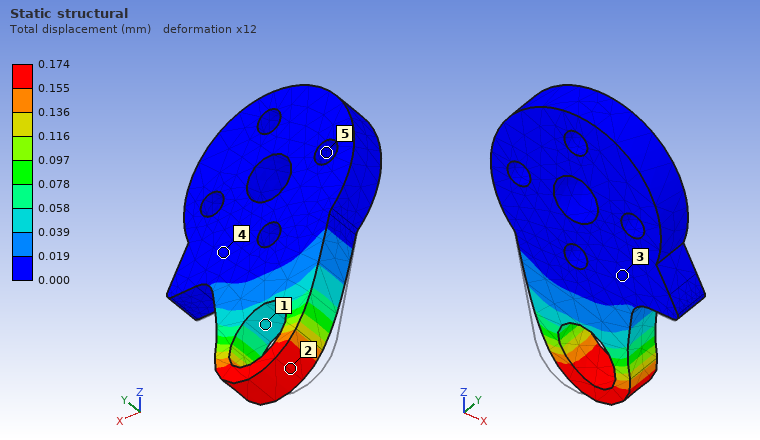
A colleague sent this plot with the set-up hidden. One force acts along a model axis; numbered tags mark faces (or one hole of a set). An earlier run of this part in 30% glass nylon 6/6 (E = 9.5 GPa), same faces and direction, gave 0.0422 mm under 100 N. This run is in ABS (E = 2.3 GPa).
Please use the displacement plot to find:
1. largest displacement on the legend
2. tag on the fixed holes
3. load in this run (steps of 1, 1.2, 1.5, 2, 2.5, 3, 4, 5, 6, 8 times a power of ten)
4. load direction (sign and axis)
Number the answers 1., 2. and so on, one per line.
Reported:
1. 0.174 mm
2. 5
3. 100 N
4. +X
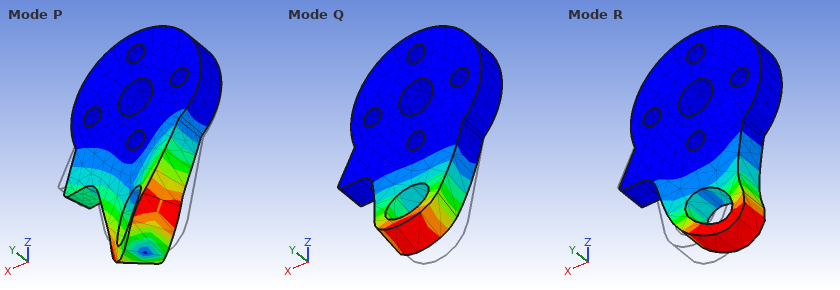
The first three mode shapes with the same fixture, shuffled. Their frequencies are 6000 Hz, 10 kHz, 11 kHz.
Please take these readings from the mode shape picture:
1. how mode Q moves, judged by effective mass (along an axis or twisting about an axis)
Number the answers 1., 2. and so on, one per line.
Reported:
1. along Y
